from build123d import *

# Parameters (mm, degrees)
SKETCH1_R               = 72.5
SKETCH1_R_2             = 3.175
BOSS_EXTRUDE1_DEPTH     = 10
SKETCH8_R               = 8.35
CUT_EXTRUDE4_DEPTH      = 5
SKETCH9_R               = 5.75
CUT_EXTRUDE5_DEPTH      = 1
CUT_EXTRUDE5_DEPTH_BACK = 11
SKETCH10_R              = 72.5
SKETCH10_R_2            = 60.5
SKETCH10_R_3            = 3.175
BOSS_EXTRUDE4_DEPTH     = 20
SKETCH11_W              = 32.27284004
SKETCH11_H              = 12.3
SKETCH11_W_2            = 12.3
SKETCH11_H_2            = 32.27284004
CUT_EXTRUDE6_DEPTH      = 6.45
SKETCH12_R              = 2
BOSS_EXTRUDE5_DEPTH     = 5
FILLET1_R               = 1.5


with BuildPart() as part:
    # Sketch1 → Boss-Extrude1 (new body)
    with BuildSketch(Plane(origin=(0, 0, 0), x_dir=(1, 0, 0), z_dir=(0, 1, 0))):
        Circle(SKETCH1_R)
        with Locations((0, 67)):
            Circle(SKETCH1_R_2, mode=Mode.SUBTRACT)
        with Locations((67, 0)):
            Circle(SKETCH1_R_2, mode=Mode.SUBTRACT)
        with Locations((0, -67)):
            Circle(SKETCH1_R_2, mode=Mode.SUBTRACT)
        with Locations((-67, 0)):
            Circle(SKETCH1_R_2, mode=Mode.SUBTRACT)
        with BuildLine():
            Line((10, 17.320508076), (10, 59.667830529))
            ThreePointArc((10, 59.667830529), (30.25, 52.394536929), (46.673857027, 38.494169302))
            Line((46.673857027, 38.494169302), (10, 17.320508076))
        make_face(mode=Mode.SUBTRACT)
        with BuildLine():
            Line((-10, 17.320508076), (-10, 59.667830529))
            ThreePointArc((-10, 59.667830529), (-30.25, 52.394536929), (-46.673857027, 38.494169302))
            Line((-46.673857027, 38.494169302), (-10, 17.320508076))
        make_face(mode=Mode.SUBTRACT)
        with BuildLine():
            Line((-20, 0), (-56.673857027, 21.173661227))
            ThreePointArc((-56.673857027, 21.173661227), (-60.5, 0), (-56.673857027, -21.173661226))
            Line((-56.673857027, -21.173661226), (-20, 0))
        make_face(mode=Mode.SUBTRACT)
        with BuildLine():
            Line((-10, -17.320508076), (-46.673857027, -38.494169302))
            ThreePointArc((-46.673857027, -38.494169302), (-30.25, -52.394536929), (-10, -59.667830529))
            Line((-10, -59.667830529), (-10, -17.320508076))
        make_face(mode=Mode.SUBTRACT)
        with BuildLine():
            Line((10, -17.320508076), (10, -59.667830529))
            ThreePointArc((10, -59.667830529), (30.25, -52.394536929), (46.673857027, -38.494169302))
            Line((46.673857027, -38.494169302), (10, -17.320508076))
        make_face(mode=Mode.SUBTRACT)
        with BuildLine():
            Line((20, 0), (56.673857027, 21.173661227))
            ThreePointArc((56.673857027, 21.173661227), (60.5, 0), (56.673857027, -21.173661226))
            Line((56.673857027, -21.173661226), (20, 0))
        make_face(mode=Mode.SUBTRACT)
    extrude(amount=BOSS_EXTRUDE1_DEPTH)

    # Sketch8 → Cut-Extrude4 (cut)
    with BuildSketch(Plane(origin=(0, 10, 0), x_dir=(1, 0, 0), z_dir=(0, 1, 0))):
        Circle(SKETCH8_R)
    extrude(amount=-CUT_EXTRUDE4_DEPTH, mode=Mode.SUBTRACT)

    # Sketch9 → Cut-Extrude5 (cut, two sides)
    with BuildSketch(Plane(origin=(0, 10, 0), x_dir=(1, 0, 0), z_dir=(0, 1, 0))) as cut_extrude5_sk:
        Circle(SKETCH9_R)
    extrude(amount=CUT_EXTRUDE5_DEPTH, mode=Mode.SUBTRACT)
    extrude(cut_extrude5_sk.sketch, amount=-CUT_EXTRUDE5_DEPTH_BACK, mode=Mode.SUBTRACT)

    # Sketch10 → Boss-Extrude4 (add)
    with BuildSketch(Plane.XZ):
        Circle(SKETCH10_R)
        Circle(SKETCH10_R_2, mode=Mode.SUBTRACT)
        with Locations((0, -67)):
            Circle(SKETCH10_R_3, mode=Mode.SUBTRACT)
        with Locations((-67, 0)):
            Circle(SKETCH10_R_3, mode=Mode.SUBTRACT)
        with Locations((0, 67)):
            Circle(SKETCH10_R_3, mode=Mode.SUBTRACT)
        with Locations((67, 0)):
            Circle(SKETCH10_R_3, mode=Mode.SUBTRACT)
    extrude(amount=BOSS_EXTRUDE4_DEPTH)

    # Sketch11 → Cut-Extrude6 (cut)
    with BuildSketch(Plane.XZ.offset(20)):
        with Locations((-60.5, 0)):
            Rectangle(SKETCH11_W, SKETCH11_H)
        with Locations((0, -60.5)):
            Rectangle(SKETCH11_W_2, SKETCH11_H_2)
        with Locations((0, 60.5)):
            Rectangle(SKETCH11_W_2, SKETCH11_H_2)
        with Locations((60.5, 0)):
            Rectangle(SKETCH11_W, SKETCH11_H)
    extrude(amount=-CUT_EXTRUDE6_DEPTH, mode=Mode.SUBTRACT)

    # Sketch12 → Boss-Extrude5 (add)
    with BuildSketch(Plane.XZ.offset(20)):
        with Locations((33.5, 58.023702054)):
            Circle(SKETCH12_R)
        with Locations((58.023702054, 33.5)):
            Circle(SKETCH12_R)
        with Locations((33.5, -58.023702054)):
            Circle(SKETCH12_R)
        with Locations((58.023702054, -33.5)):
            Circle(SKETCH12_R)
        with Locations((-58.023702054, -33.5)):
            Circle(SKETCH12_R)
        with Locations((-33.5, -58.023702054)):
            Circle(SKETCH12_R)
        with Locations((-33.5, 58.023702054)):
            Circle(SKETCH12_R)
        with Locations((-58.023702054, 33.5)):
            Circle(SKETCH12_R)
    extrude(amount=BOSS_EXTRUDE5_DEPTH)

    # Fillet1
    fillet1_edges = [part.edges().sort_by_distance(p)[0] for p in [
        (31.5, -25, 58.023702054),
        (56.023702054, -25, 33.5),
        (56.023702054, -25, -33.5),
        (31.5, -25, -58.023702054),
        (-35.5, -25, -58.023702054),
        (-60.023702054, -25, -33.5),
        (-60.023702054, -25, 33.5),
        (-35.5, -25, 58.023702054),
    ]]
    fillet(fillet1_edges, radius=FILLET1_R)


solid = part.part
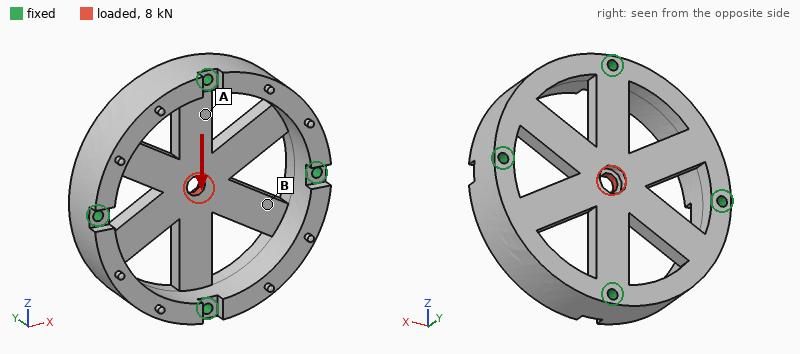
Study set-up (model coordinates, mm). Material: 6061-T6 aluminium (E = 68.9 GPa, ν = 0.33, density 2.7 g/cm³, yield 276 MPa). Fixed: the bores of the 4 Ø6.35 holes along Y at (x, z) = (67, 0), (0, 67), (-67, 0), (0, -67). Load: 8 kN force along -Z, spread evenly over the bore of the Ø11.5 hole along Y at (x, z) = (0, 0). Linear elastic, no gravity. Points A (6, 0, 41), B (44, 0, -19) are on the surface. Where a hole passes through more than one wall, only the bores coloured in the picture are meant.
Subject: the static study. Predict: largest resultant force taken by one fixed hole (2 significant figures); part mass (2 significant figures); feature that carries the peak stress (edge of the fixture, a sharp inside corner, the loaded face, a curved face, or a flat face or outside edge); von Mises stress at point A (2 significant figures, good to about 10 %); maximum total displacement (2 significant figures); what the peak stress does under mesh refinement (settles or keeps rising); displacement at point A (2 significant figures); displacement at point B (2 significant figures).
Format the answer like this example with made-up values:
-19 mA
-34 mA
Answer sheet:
2.8 kN
550 g
a sharp inside corner
19 MPa
20 µm
keeps rising
7.3 µm
6.0 µm
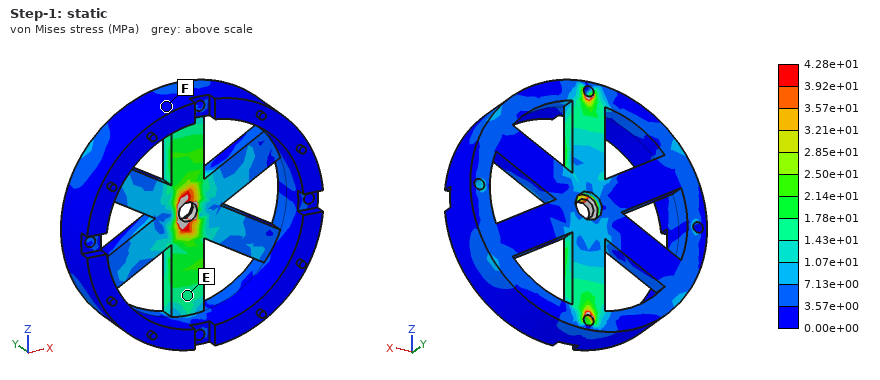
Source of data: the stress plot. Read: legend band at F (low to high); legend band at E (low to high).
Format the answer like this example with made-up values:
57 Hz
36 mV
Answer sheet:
0.00e+00 to 3.57e+00 MPa
1.43e+01 to 1.78e+01 MPa
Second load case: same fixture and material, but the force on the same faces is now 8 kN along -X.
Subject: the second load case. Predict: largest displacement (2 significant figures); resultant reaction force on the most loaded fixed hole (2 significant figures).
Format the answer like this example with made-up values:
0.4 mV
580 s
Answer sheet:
32 µm
2.8 kN
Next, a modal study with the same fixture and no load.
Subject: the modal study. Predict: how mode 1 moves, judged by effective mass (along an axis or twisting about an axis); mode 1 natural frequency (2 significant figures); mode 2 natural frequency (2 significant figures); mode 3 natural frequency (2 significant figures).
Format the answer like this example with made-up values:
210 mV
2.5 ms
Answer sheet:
along Y
3700 Hz
7100 Hz
7400 Hz
